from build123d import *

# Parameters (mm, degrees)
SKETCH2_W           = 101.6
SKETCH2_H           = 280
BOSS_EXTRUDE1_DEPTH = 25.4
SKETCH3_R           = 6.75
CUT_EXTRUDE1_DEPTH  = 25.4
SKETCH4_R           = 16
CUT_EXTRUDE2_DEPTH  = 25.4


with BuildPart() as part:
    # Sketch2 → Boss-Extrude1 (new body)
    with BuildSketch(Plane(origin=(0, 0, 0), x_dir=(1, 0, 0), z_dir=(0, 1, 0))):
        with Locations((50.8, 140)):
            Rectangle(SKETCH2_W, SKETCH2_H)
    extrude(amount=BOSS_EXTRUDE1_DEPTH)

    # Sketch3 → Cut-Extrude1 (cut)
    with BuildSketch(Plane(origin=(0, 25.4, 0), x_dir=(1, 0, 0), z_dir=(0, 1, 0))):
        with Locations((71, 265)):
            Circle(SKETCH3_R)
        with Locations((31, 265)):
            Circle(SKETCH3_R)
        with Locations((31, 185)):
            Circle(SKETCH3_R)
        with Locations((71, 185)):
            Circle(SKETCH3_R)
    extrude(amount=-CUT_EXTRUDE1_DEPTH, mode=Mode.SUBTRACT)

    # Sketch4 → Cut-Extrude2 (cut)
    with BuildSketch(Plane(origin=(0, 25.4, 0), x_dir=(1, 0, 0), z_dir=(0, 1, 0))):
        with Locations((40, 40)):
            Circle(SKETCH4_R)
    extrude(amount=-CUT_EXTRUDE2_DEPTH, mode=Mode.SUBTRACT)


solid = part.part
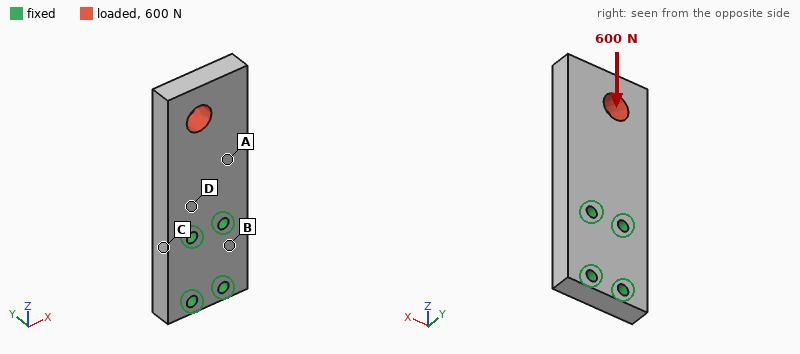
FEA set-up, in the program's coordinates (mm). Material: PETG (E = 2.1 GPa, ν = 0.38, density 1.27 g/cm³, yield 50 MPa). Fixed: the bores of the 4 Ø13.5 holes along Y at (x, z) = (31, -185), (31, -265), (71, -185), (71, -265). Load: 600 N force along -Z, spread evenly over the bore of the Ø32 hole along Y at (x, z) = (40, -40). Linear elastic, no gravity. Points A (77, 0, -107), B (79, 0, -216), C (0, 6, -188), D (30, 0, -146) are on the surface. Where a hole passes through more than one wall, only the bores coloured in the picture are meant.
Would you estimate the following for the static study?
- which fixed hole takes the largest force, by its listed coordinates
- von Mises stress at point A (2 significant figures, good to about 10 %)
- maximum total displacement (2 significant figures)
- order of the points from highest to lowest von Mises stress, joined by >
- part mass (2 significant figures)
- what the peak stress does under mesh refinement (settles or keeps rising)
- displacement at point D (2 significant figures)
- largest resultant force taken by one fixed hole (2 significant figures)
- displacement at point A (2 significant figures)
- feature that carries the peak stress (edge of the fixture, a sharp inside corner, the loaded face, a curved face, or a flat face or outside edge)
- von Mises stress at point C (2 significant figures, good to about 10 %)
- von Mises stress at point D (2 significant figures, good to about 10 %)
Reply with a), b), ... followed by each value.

a) (31, -185)
b) 0.16 MPa
c) 37 µm
d) D > C > A > B
e) 870 g
f) keeps rising
g) 7.0 µm
h) 370 N
i) 7.6 µm
j) edge of the fixture
k) 0.25 MPa
l) 0.33 MPa
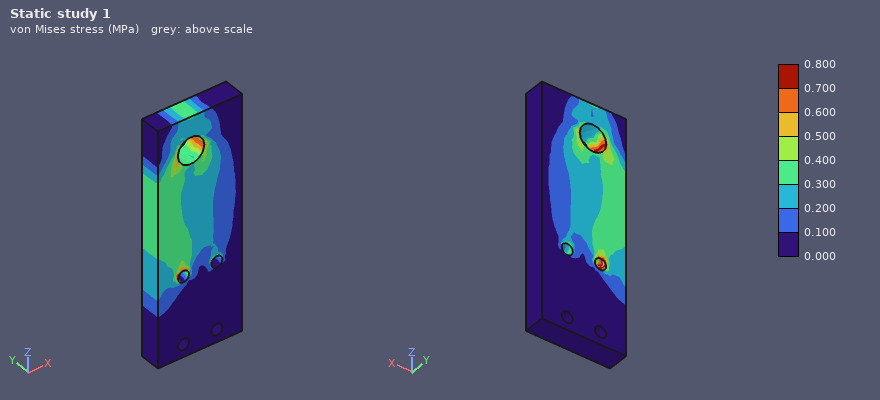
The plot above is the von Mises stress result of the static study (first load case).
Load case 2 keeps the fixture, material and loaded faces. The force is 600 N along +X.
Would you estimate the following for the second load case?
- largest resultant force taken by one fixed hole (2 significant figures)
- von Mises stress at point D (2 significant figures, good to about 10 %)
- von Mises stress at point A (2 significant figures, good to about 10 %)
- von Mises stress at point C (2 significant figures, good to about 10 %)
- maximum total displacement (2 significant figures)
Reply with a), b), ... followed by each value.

a) 1.3 kN
b) 0.89 MPa
c) 0.64 MPa
d) 1.4 MPa
e) 0.32 mm
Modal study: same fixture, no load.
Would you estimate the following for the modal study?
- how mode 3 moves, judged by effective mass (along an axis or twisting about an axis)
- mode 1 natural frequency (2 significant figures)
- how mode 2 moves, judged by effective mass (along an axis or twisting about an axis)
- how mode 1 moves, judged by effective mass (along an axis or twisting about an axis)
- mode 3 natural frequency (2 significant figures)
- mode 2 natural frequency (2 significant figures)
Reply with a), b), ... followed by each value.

a) twisting about Z
b) 160 Hz
c) along X
d) along Y
e) 510 Hz
f) 460 Hz
